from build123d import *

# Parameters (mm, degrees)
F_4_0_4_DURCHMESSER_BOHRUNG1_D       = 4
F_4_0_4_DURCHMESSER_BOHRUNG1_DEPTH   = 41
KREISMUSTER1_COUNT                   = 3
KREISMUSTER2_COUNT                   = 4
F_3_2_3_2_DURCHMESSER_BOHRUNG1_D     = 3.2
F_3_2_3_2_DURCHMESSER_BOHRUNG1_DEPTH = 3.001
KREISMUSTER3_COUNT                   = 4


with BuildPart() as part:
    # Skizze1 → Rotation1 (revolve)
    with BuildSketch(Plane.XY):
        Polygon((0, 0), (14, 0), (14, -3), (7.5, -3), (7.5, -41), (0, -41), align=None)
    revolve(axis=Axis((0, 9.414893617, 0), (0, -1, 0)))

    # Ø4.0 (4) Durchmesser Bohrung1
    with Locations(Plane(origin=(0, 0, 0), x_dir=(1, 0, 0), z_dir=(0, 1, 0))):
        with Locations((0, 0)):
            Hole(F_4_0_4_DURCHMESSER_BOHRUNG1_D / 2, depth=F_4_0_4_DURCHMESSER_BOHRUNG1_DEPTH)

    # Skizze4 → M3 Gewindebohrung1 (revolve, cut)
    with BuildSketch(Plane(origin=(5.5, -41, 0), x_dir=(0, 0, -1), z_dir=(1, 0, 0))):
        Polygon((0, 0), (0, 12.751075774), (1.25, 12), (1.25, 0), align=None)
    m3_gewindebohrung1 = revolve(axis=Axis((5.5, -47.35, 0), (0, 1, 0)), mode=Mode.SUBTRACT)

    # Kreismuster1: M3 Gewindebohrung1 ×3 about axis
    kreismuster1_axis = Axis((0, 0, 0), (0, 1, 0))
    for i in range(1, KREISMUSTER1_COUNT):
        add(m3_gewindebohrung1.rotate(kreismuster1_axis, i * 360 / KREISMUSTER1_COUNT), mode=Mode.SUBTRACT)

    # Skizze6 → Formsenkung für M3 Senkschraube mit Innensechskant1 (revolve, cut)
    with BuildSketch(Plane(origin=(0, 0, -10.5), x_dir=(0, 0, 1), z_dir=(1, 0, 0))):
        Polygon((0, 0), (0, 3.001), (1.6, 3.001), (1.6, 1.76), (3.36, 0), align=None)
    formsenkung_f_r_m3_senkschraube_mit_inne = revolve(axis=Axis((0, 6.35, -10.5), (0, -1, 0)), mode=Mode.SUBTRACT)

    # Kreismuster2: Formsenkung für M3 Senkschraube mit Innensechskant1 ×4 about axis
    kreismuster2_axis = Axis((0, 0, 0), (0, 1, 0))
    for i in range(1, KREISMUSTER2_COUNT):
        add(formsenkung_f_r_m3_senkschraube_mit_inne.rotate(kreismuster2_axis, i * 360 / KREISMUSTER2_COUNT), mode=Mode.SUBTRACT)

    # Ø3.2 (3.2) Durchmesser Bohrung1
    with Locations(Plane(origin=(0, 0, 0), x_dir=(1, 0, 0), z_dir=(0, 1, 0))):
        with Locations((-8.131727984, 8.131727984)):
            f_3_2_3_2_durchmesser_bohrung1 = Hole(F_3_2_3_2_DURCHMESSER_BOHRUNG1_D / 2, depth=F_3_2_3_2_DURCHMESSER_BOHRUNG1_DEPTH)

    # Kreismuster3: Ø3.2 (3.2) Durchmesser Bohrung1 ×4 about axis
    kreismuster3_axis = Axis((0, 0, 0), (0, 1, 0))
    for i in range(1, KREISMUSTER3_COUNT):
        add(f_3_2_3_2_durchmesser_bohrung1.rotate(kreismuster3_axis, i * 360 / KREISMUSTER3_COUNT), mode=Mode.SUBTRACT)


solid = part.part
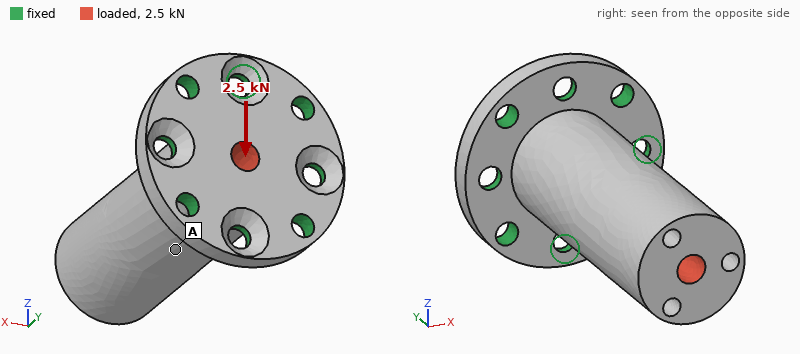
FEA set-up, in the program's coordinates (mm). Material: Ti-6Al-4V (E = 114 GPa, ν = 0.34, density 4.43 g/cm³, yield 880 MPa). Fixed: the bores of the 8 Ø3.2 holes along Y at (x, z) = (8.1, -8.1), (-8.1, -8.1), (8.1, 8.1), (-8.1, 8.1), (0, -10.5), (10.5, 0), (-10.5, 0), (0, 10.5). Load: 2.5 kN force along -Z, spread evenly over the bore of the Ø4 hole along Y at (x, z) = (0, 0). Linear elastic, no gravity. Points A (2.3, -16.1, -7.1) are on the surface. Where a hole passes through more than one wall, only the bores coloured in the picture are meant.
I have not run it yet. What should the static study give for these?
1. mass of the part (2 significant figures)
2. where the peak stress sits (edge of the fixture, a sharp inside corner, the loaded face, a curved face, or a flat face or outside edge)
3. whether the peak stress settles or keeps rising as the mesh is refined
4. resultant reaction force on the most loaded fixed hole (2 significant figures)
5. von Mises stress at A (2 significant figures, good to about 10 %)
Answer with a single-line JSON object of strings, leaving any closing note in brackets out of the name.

{"mass of the part": "34 g", "where the peak stress sits": "edge of the fixture", "whether the peak stress settles or keeps rising as the mesh is refined": "keeps rising", "resultant reaction force on the most loaded fixed hole": "1.3 kN", "von Mises stress at A": "54 MPa"}
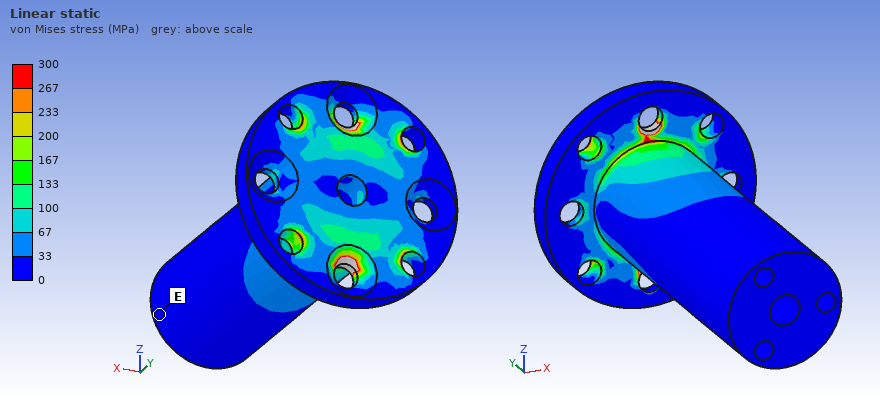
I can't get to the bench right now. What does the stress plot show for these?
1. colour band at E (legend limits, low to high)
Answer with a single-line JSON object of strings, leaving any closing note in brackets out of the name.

{"colour band at E": "0 to 33 MPa"}
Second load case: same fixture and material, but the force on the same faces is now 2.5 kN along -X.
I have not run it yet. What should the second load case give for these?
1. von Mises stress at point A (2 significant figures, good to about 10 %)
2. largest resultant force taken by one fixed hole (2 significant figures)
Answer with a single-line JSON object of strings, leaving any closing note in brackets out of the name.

{"von Mises stress at point A": "27 MPa", "largest resultant force taken by one fixed hole": "1.3 kN"}
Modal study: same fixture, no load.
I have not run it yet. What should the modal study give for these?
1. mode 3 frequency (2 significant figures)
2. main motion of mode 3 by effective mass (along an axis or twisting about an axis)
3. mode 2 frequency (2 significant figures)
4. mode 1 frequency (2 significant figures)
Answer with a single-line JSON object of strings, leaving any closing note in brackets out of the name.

{"mode 3 frequency": "20 kHz", "main motion of mode 3 by effective mass": "twisting about Y", "mode 2 frequency": "5300 Hz", "mode 1 frequency": "5300 Hz"}
